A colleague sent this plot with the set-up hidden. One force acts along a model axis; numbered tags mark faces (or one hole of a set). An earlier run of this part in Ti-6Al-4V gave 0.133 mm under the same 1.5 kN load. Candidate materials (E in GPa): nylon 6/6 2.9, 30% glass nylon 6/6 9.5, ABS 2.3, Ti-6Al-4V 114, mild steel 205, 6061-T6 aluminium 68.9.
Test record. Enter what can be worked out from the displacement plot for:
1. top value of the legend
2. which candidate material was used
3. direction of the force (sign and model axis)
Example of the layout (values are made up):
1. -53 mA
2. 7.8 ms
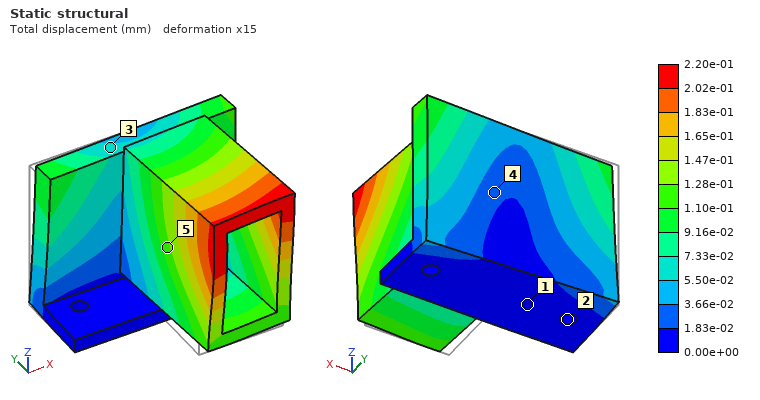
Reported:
1. 2.20e-01 mm
2. 6061-T6 aluminium
3. +X
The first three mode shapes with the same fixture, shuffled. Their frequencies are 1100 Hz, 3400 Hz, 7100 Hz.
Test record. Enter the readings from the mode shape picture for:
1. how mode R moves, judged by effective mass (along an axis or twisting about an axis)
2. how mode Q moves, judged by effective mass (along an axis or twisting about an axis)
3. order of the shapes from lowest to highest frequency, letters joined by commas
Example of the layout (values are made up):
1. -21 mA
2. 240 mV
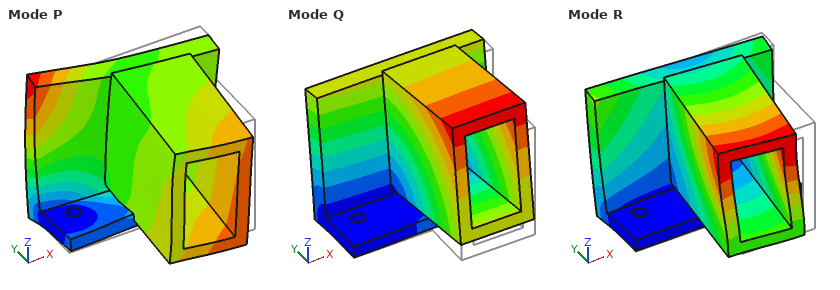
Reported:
1. along X
2. along Y
3. Q, R, P
